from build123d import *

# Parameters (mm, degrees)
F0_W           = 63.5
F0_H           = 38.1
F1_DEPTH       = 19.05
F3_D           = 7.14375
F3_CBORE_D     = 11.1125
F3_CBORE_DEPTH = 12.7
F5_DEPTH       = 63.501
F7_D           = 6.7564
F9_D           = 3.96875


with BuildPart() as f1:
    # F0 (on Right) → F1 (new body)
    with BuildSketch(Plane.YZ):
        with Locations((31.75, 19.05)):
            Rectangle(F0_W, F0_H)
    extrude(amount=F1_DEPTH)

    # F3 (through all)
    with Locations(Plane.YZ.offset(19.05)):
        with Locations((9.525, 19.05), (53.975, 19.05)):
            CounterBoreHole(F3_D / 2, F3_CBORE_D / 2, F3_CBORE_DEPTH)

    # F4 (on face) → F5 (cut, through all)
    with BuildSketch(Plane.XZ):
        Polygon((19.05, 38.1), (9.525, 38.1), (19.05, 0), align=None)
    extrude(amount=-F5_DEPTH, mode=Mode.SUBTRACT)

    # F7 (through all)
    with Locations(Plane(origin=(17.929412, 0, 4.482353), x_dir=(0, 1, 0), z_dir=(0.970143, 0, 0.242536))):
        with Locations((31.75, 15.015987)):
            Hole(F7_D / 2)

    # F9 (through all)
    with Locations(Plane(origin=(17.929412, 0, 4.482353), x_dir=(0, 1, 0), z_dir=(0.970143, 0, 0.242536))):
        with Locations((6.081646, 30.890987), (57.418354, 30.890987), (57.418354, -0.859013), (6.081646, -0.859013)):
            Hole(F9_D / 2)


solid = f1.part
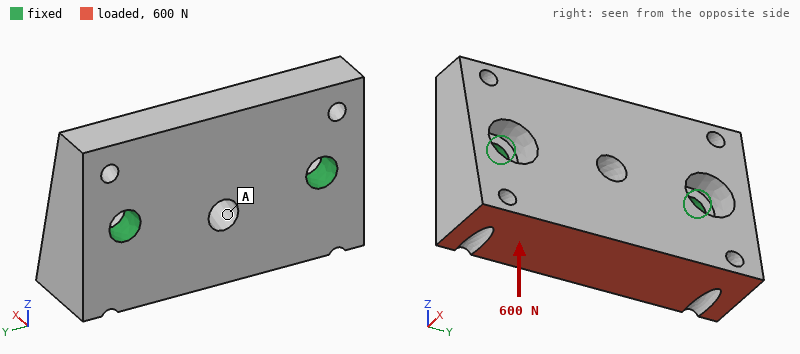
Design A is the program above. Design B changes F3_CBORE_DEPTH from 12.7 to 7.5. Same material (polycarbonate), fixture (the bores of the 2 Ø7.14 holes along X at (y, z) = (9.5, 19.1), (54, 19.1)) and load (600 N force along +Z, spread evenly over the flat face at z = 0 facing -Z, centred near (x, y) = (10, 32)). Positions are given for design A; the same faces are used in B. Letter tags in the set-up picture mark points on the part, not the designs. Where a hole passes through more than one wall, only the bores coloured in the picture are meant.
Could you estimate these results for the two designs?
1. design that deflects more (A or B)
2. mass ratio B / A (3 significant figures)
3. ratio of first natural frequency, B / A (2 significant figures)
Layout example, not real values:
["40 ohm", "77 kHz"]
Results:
["A", "1.02", "1.7"]
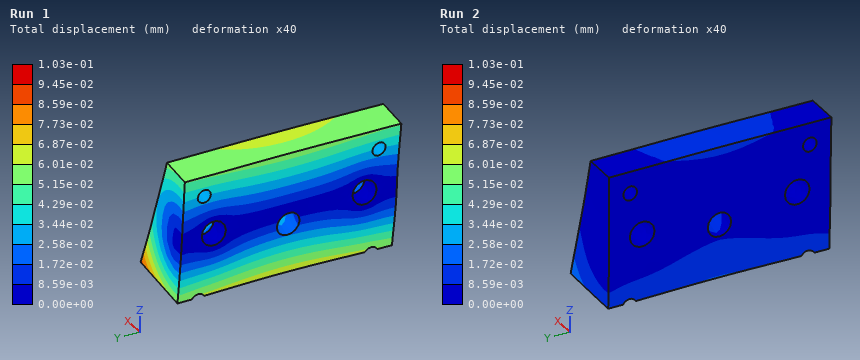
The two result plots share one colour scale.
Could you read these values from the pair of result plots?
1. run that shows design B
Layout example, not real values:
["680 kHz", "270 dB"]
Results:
["Run 2"]
